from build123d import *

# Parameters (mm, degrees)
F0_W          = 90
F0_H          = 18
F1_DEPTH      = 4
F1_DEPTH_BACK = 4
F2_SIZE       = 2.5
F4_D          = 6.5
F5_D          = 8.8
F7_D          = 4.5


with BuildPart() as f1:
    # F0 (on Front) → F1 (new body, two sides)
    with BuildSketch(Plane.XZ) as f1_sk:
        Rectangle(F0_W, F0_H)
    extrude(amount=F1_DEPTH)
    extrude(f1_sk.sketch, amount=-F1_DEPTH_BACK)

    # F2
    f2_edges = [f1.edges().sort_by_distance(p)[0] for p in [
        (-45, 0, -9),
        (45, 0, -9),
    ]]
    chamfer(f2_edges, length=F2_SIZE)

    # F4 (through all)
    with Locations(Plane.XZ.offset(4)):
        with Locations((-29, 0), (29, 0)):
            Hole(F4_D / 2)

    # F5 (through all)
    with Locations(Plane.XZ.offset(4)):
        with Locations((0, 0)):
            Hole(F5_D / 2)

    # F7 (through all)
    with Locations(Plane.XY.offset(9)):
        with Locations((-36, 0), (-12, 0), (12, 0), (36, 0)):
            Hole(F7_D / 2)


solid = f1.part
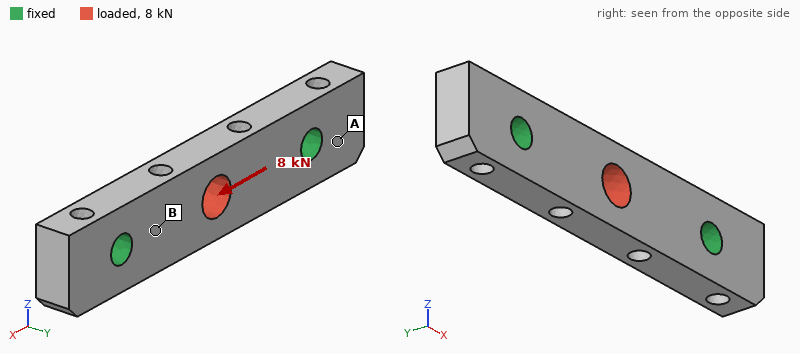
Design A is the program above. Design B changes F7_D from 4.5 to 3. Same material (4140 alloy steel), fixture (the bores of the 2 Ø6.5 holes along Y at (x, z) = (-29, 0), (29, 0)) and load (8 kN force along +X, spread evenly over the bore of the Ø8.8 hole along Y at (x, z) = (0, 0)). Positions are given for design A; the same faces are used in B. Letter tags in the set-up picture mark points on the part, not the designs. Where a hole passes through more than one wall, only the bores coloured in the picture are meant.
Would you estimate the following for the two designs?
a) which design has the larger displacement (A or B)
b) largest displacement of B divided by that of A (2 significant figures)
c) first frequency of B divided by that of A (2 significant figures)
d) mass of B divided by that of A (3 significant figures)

A
0.86
1.0
1.06
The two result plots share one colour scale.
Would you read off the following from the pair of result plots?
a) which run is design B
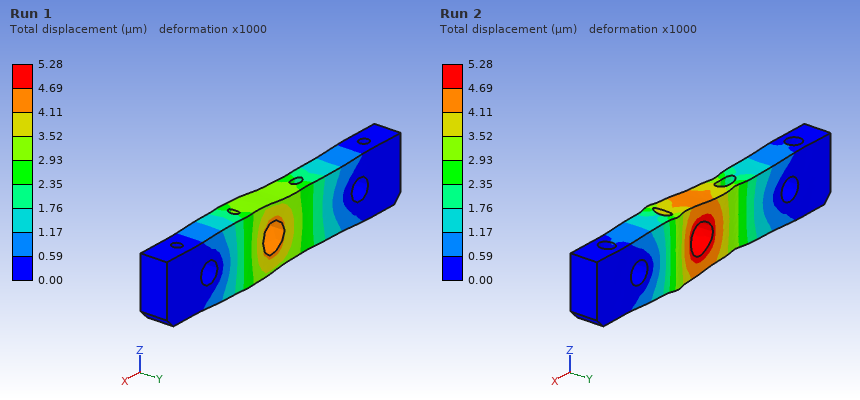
Run 1
